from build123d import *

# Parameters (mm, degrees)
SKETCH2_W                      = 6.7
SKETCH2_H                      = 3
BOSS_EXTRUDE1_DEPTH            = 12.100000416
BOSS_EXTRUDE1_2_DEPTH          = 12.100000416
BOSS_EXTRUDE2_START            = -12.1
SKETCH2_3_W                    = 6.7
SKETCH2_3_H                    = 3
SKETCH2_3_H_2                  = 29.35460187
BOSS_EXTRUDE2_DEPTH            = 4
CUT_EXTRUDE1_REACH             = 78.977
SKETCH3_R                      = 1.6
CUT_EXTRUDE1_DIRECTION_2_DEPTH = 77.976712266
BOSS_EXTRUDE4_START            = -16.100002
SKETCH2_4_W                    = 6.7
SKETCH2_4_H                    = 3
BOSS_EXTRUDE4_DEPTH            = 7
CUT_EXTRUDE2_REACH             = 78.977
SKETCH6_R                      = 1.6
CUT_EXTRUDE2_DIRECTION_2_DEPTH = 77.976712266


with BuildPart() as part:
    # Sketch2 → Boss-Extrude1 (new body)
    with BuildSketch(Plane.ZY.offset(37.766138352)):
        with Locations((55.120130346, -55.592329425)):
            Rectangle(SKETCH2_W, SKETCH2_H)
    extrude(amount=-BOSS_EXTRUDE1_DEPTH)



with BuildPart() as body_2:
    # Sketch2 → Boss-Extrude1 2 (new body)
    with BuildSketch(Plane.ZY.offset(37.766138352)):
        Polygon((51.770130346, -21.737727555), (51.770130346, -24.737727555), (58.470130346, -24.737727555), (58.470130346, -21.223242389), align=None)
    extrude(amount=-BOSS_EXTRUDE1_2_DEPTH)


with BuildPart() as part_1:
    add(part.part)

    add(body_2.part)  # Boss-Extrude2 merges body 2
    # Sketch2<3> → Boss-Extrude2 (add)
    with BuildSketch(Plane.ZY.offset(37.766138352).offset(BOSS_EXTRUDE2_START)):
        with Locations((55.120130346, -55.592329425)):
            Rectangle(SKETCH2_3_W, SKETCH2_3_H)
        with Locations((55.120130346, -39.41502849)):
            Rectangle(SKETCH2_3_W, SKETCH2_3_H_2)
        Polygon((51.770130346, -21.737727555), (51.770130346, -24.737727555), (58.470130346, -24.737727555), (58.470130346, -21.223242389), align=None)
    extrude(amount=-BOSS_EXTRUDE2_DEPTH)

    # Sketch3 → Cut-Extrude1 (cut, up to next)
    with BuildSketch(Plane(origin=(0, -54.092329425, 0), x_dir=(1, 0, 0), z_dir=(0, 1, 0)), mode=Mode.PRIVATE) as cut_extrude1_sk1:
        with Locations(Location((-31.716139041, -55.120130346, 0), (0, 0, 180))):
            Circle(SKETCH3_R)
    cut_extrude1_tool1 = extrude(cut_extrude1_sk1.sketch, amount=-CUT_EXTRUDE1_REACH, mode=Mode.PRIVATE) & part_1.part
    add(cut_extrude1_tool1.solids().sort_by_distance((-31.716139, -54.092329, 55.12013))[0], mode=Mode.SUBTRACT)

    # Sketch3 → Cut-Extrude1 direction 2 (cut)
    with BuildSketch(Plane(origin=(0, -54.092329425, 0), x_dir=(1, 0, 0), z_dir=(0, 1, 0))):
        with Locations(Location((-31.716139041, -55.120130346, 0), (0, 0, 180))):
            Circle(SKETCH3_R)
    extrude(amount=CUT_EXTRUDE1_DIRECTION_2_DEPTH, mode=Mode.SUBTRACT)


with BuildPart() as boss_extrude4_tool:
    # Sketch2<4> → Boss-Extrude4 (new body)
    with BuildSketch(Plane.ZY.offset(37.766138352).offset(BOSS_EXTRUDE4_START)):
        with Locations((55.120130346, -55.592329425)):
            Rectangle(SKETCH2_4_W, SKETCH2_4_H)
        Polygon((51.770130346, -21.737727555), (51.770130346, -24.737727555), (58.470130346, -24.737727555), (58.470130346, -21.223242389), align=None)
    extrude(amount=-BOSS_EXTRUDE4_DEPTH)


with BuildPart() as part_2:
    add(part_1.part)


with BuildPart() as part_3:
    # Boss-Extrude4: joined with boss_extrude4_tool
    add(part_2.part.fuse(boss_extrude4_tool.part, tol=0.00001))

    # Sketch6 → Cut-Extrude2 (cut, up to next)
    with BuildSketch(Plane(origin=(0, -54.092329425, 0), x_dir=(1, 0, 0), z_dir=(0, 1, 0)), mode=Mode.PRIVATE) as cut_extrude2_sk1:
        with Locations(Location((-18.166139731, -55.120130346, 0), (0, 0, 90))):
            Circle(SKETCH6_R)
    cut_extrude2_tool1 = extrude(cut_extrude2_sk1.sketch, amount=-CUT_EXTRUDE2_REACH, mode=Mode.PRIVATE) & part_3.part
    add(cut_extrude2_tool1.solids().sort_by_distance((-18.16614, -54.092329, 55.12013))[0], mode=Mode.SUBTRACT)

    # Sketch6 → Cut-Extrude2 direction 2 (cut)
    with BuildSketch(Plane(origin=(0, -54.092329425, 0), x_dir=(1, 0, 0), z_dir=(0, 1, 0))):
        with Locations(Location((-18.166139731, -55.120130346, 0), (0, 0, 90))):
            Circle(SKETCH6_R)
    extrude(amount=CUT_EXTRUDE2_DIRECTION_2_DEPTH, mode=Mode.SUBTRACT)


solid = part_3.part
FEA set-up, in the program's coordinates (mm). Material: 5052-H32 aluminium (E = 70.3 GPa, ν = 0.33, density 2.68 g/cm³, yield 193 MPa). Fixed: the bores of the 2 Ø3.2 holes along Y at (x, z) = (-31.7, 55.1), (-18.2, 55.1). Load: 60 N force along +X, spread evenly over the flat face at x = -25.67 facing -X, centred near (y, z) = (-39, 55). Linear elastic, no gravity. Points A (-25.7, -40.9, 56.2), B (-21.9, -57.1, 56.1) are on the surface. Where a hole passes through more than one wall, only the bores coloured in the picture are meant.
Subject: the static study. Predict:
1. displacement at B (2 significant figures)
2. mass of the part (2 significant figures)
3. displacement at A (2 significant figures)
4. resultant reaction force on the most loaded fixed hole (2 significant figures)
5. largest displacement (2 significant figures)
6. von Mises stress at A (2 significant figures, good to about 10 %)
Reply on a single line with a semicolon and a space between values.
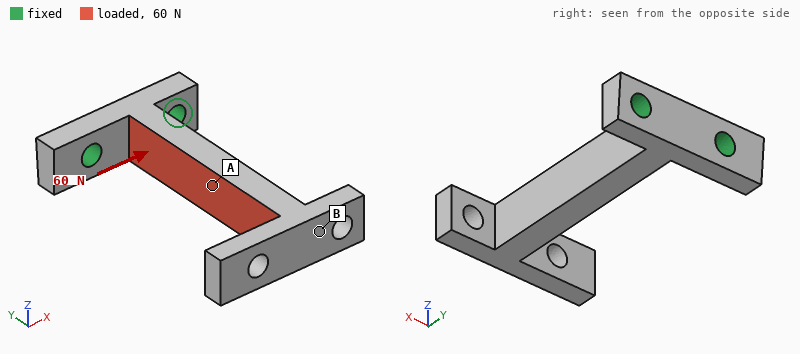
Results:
0.11 mm; 4.4 g; 0.045 mm; 110 N; 0.13 mm; 10 MPa
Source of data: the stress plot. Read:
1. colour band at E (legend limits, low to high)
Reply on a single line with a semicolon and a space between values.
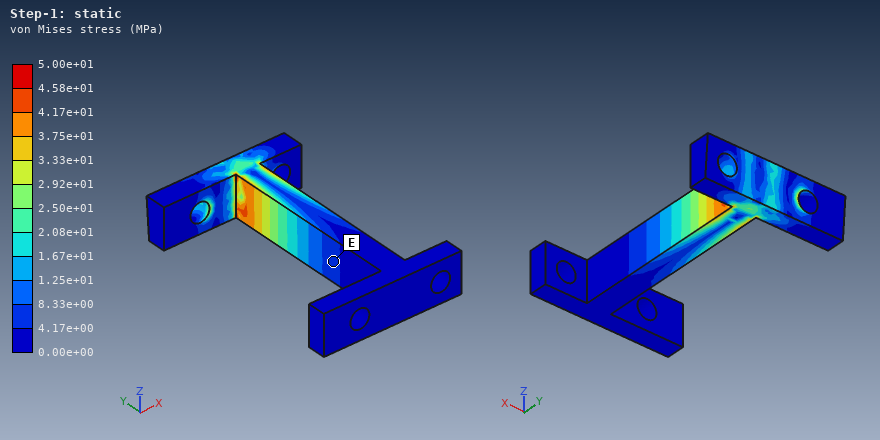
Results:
4.17e+00 to 8.33e+00 MPa
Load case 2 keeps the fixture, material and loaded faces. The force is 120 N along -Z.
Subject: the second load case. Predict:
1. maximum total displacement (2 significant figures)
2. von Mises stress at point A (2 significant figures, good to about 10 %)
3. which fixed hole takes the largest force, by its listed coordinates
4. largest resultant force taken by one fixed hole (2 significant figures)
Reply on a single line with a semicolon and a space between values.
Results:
0.17 mm; 13 MPa; (-18.2, 55.1); 66 N
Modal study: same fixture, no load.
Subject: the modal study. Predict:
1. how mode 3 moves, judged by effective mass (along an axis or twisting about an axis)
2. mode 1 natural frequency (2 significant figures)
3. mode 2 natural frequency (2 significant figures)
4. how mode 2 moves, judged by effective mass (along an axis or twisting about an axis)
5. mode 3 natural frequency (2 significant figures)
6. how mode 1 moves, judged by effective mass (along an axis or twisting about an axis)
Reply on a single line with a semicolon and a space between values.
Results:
twisting about Y; 1800 Hz; 2300 Hz; along Z; 5700 Hz; along X
